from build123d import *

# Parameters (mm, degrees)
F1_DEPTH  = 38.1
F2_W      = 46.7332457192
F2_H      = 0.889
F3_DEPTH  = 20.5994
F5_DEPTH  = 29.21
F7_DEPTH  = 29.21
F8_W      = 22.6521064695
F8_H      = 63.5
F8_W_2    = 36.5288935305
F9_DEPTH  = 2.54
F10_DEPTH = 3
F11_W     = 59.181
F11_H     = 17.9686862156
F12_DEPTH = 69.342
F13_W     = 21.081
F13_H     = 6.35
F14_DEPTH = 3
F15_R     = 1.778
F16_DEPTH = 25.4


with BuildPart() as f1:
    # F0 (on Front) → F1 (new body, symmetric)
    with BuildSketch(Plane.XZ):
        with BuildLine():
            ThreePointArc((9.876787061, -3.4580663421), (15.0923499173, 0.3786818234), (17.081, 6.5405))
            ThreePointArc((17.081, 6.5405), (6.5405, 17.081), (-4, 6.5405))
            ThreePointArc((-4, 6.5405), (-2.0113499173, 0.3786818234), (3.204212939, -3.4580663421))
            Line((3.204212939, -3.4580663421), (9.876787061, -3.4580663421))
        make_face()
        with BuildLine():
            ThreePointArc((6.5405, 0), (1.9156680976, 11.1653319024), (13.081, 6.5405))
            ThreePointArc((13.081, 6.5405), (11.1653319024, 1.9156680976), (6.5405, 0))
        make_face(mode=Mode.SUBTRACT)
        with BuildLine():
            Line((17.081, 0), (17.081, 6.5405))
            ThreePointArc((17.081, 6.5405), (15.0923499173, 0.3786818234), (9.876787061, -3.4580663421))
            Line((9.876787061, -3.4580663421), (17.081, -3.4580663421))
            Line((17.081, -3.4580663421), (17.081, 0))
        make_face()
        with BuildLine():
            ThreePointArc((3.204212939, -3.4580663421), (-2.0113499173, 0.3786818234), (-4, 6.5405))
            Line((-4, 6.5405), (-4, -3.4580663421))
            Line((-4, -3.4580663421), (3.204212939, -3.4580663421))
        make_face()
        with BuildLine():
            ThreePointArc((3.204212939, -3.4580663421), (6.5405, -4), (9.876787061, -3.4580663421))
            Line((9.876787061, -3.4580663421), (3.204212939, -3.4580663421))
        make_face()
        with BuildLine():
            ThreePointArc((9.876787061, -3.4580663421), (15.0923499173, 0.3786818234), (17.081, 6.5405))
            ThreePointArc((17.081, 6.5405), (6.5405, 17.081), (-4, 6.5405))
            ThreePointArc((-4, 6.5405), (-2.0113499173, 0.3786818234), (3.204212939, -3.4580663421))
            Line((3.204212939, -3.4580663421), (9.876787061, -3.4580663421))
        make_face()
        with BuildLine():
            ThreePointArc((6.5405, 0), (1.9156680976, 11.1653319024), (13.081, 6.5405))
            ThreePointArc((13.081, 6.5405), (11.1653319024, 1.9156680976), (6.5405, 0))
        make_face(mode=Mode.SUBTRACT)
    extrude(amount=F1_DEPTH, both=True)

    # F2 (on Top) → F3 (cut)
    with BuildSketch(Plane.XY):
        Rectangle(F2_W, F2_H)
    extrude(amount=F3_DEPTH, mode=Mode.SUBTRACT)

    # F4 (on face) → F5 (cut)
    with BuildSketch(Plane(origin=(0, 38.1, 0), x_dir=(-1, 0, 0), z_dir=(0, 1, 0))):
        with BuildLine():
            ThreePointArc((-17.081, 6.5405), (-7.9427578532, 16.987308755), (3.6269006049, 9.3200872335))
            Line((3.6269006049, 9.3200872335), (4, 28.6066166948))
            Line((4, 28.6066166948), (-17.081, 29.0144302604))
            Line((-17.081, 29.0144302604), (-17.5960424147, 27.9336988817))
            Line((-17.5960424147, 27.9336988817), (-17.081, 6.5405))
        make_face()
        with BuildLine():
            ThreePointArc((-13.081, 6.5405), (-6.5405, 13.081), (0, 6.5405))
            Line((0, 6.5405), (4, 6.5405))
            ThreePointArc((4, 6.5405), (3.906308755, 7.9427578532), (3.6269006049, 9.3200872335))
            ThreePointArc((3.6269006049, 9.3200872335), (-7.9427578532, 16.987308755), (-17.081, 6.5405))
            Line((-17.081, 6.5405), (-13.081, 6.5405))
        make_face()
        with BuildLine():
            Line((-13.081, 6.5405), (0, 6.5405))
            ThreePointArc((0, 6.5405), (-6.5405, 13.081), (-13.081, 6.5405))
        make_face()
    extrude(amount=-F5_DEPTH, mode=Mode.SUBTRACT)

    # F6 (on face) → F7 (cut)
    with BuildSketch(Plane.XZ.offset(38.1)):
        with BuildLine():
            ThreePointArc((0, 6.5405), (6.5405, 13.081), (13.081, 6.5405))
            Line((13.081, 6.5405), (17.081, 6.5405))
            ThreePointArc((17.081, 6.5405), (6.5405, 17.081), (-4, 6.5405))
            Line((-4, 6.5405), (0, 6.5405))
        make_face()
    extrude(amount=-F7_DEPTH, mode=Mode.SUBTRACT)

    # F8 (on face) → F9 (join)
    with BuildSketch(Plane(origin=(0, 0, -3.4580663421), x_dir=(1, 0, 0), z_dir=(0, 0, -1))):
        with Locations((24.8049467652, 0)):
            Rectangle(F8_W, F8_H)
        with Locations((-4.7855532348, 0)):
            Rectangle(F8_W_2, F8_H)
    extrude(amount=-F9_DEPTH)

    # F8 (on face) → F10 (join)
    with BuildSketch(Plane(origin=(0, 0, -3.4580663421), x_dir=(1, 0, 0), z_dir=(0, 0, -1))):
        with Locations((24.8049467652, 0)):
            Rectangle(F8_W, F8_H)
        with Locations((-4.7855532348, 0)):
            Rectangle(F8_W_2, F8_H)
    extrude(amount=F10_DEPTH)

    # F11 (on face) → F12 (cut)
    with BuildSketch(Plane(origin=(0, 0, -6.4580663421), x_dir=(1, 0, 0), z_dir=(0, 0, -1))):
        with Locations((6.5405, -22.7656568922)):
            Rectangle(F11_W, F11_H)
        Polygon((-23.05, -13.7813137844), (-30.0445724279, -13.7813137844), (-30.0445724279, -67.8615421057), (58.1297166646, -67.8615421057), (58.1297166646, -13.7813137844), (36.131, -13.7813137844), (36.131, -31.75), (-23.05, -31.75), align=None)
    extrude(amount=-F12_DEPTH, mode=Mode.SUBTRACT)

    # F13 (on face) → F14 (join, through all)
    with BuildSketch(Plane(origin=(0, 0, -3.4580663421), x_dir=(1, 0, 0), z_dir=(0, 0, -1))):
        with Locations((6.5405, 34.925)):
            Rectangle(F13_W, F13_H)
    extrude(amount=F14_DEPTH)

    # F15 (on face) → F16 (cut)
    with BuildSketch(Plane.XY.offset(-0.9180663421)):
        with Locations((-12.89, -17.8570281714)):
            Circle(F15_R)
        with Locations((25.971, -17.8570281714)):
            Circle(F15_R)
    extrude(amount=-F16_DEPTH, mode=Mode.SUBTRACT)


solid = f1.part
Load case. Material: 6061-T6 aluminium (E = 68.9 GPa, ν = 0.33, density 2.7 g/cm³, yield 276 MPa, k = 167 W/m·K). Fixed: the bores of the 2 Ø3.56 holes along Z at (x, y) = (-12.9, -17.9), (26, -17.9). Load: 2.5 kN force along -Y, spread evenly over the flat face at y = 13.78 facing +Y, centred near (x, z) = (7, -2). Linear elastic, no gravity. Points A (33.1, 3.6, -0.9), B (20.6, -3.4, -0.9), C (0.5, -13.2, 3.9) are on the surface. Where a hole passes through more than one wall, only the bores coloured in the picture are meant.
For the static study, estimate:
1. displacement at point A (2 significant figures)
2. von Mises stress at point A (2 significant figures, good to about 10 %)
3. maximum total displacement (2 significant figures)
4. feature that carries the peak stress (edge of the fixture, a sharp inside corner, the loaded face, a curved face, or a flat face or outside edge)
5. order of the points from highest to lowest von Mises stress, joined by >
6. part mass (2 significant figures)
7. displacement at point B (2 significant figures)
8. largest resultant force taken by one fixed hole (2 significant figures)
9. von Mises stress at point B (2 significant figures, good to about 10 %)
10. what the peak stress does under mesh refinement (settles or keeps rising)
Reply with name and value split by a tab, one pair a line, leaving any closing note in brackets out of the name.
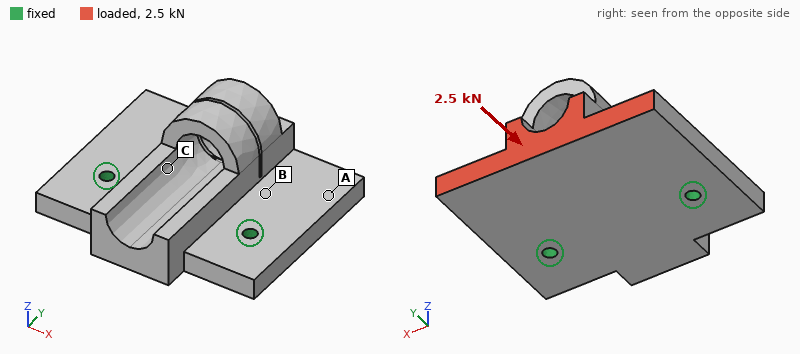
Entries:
displacement at point A	9.7 µm
von Mises stress at point A	8.7 MPa
maximum total displacement	26 µm
feature that carries the peak stress	edge of the fixture
order of the points from highest to lowest von Mises stress, joined by >	B > A > C
part mass	59 g
displacement at point B	7.2 µm
largest resultant force taken by one fixed hole	1.3 kN
von Mises stress at point B	12 MPa
what the peak stress does under mesh refinement	keeps rising
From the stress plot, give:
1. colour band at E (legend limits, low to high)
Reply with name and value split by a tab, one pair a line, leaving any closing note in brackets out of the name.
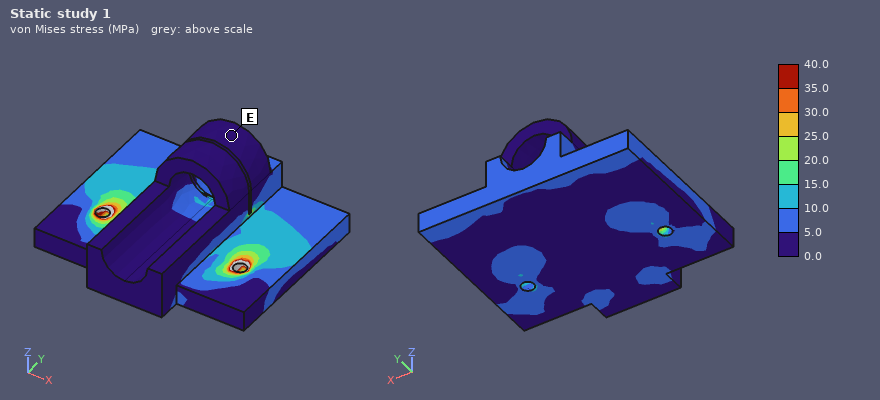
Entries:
colour band at E	0.0 to 5.0 MPa
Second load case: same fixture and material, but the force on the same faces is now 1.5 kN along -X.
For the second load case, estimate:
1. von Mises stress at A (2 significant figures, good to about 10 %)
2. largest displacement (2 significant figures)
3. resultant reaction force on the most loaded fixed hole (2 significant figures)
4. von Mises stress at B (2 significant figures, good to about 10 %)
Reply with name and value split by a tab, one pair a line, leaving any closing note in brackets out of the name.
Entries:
von Mises stress at A	4.8 MPa
largest displacement	13 µm
resultant reaction force on the most loaded fixed hole	1.4 kN
von Mises stress at B	12 MPa
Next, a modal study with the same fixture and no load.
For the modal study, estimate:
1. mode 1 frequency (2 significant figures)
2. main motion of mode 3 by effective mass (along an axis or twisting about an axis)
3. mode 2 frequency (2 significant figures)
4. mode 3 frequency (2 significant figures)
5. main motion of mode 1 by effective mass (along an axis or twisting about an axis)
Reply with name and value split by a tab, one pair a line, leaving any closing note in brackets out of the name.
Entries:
mode 1 frequency	3200 Hz
main motion of mode 3 by effective mass	along Z
mode 2 frequency	7100 Hz
mode 3 frequency	9700 Hz
main motion of mode 1 by effective mass	along Z
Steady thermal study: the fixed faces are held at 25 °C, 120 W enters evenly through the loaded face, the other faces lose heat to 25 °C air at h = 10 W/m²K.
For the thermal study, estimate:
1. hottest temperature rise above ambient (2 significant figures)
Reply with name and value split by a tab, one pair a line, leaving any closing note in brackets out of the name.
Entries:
hottest temperature rise above ambient	72 K
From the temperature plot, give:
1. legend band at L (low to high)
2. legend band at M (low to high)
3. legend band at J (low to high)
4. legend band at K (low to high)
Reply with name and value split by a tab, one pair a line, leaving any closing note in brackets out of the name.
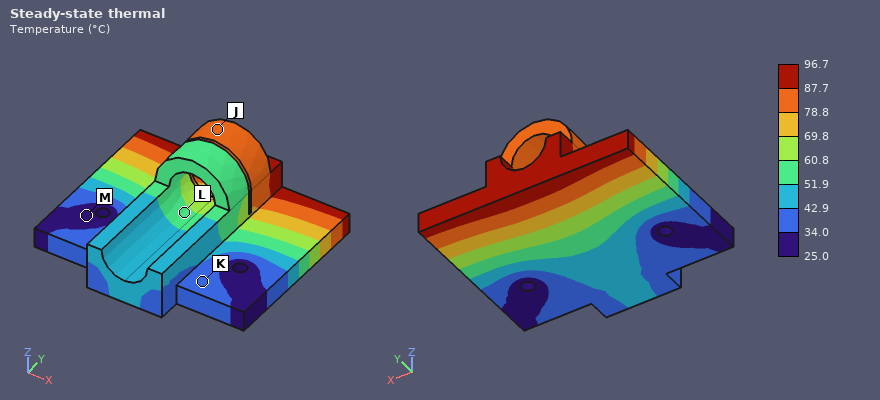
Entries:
legend band at L	51.9 to 60.8 °C
legend band at M	25.0 to 34.0 °C
legend band at J	78.8 to 87.7 °C
legend band at K	34.0 to 42.9 °C
